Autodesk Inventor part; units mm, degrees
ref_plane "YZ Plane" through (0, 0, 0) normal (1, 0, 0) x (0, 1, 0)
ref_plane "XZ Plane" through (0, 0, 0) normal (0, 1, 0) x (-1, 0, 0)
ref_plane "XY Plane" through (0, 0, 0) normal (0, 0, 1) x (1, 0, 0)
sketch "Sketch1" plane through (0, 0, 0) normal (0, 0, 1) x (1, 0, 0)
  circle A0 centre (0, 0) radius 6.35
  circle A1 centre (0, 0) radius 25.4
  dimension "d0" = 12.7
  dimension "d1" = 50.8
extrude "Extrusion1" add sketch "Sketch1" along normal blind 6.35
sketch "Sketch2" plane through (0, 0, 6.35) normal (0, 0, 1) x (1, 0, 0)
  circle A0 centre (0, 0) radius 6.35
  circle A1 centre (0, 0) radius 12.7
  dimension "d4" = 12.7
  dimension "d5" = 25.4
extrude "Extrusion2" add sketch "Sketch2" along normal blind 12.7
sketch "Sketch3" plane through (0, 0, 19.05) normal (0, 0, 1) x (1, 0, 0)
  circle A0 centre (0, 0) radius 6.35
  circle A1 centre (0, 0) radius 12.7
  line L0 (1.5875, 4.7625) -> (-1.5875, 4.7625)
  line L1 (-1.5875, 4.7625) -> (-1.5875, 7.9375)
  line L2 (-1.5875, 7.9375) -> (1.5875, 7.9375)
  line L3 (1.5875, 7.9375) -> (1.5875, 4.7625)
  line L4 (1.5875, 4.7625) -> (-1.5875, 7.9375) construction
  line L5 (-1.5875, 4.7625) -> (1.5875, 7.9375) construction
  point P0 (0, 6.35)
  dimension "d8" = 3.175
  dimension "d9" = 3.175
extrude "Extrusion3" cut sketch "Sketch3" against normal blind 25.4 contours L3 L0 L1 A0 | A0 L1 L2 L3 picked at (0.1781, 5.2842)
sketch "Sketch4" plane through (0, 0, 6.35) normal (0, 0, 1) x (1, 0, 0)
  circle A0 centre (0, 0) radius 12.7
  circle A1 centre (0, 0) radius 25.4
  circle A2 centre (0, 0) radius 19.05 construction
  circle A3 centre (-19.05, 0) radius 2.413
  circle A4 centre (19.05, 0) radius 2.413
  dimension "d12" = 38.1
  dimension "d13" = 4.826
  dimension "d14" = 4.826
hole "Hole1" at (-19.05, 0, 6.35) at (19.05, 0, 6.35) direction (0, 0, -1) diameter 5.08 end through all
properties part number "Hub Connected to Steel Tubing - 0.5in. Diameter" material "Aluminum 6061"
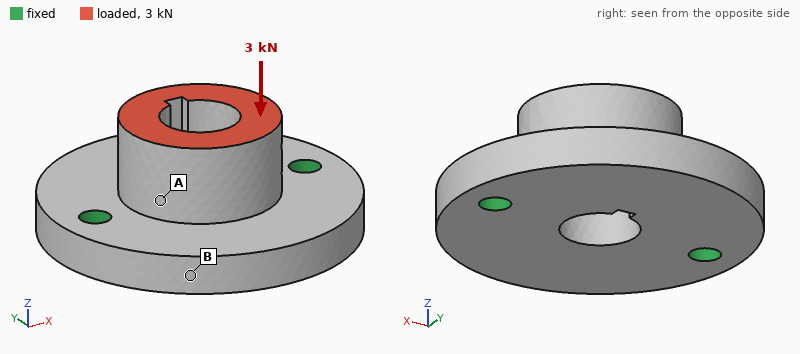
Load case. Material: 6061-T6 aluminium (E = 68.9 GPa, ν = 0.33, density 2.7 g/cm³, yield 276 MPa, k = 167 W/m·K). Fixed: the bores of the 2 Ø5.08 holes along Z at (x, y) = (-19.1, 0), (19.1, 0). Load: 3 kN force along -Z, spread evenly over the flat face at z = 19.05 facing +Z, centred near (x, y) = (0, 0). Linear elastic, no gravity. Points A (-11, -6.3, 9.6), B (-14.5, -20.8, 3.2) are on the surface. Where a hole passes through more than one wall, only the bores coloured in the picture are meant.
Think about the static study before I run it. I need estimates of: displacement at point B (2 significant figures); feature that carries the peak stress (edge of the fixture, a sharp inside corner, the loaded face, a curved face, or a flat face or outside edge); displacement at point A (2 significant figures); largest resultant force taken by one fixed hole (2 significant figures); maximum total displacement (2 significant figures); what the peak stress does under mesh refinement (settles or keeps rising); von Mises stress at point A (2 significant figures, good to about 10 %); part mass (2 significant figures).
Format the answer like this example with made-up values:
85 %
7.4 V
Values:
10 µm
edge of the fixture
10 µm
1.6 kN
16 µm
keeps rising
21 MPa
45 g
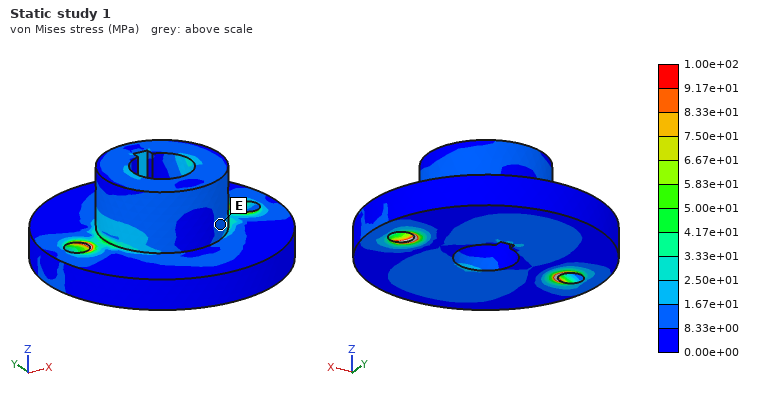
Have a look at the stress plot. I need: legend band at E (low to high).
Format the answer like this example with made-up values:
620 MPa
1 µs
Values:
8.33e+00 to 1.67e+01 MPa
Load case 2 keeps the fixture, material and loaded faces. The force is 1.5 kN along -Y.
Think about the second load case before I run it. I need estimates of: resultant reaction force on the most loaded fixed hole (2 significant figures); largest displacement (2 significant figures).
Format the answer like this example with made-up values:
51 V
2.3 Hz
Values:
750 N
49 µm
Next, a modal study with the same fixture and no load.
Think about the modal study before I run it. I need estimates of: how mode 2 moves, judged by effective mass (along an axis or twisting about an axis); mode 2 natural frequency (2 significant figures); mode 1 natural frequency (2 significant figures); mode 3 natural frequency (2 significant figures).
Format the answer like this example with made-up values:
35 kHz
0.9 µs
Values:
along Z
12 kHz
6700 Hz
20 kHz
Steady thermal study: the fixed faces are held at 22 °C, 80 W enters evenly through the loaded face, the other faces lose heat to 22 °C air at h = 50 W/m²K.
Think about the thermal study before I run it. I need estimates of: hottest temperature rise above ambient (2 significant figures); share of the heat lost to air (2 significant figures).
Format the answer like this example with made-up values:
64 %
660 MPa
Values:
33 K
5.5 %
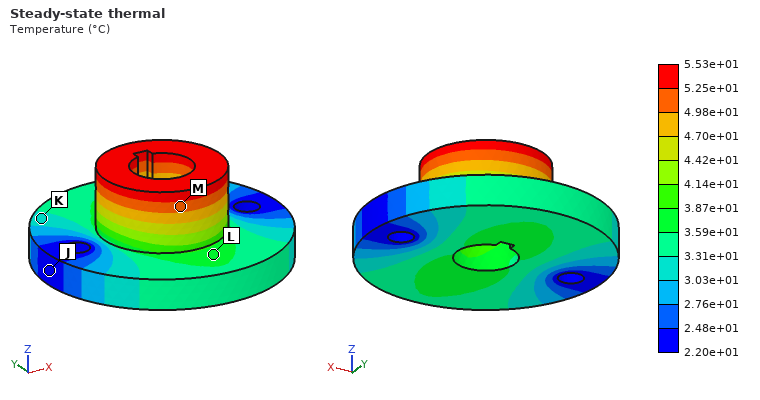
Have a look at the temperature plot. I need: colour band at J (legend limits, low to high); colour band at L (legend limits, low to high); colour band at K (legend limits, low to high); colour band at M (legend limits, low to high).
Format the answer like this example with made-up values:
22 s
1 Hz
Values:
2.20e+01 to 2.48e+01 °C
3.59e+01 to 3.87e+01 °C
3.03e+01 to 3.31e+01 °C
4.98e+01 to 5.25e+01 °C
